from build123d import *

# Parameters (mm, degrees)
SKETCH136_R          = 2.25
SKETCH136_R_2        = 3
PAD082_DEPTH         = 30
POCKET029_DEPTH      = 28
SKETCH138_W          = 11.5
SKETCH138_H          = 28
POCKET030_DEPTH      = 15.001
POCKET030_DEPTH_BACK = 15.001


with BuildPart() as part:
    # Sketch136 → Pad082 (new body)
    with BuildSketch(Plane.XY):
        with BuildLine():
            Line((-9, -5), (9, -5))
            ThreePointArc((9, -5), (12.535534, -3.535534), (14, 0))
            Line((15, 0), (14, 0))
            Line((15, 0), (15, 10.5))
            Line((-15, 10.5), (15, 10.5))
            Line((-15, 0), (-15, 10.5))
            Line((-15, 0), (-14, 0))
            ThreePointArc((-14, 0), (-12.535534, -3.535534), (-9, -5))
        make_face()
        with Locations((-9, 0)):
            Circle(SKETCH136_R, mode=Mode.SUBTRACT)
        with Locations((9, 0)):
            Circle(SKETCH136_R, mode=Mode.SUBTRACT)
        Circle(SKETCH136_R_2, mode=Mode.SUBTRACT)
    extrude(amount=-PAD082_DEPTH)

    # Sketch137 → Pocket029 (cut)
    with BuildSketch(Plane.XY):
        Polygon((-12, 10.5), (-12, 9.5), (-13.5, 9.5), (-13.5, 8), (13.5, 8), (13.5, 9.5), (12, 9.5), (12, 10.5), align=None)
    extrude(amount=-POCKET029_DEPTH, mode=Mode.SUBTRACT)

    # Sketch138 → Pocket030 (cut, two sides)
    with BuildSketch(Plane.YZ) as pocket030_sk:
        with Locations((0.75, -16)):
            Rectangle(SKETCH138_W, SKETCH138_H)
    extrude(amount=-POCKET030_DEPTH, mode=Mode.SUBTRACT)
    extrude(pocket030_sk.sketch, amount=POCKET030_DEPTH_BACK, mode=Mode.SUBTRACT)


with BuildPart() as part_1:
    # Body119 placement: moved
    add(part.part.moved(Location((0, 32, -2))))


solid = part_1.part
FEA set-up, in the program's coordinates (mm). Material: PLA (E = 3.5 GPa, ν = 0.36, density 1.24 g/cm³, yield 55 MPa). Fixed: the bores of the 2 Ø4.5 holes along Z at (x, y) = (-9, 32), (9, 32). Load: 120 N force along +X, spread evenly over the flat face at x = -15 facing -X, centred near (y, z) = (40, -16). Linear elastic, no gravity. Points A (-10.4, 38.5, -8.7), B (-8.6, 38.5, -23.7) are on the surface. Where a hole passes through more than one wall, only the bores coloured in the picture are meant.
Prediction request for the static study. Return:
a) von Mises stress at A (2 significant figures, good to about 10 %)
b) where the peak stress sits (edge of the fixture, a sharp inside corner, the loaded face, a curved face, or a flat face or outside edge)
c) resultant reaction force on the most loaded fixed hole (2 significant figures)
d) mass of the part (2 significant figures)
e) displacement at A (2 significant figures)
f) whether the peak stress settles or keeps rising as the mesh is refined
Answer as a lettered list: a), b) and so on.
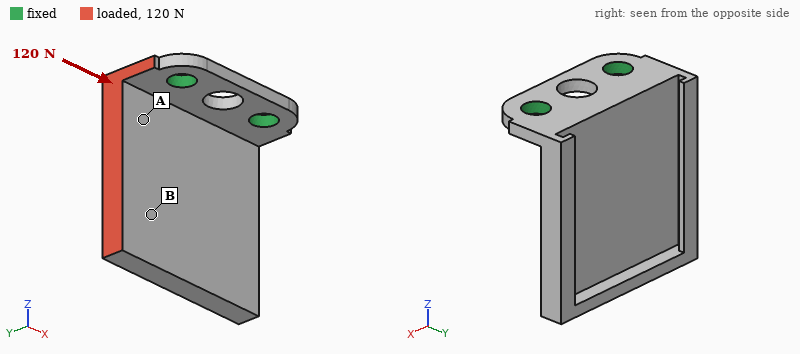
a) 10 MPa
b) edge of the fixture
c) 100 N
d) 2.9 g
e) 0.17 mm
f) keeps rising
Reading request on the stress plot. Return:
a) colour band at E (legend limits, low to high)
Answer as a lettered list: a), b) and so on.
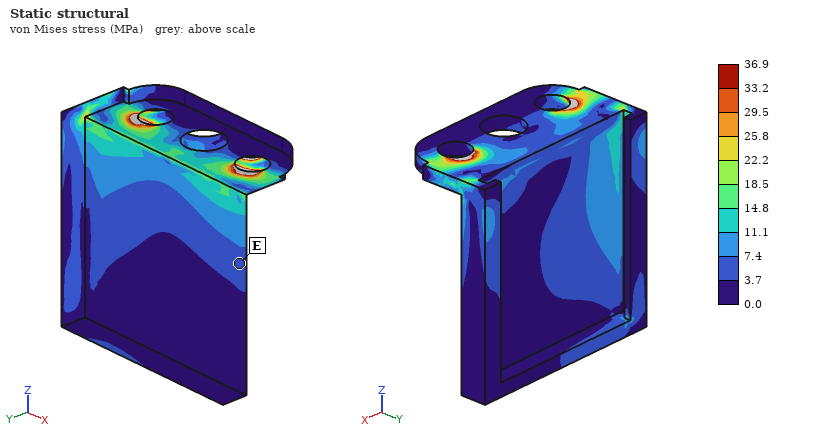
a) 3.7 to 7.4 MPa
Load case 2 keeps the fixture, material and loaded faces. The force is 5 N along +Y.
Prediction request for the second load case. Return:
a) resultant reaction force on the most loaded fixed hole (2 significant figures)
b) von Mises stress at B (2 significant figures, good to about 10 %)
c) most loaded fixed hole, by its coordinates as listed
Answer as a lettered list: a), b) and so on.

a) 5.8 N
b) 0.96 MPa
c) (-9, 32)
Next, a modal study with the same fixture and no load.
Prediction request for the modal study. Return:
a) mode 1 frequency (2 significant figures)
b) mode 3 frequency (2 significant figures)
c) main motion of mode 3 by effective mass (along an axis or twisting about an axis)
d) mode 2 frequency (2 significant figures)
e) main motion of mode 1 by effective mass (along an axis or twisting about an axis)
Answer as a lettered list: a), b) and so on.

a) 460 Hz
b) 1800 Hz
c) along X
d) 1000 Hz
e) along Y
